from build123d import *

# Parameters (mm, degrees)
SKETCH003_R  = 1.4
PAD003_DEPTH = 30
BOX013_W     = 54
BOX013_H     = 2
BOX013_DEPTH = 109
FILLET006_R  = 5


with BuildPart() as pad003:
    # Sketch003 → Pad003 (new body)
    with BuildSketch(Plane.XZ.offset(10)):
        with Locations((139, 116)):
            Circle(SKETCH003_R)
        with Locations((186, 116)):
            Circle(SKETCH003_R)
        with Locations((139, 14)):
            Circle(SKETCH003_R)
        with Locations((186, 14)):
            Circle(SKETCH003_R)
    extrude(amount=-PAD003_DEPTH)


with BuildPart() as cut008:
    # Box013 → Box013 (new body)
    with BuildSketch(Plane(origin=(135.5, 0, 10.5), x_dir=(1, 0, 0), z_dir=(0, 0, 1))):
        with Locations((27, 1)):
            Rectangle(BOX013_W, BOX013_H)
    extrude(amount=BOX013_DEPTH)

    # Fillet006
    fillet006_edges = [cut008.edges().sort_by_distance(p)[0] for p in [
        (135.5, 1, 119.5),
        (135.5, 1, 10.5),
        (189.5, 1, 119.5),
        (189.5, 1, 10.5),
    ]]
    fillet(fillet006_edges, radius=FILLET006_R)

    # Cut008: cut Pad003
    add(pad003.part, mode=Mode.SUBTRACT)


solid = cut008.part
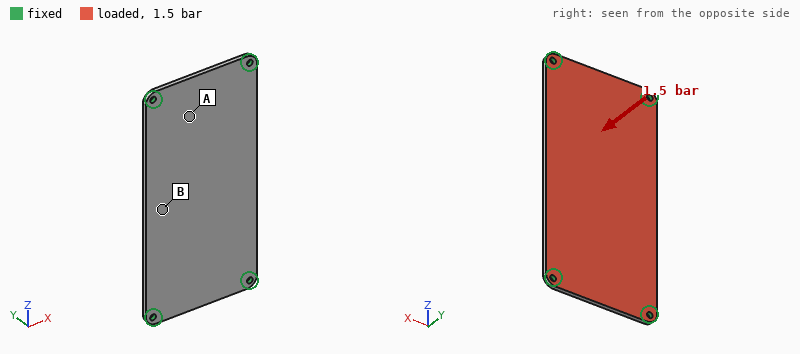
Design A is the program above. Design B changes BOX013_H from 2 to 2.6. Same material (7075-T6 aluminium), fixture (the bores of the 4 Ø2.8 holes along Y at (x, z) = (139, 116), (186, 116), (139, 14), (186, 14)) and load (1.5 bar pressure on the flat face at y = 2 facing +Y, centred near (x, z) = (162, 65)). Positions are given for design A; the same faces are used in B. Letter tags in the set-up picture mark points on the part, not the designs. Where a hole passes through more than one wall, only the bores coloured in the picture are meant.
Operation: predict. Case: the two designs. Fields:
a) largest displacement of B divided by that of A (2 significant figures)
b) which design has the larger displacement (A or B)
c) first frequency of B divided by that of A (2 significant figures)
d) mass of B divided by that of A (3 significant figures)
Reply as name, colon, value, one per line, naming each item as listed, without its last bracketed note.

largest displacement of B divided by that of A: 0.47
which design has the larger displacement: A
first frequency of B divided by that of A: 1.3
mass of B divided by that of A: 1.30
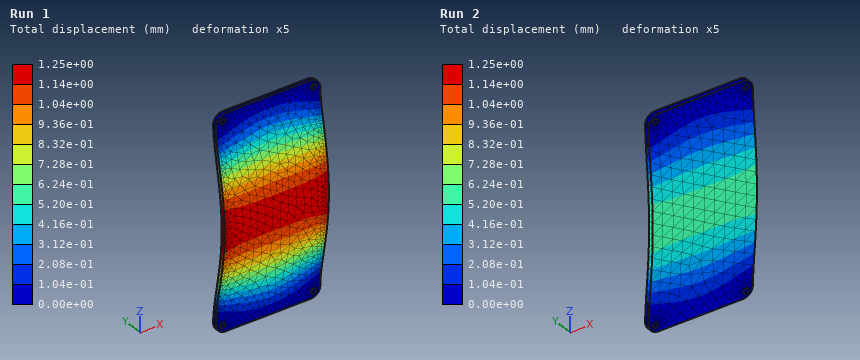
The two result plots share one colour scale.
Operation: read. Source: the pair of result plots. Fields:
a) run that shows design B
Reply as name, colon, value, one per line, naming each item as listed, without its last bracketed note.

run that shows design B: Run 2
